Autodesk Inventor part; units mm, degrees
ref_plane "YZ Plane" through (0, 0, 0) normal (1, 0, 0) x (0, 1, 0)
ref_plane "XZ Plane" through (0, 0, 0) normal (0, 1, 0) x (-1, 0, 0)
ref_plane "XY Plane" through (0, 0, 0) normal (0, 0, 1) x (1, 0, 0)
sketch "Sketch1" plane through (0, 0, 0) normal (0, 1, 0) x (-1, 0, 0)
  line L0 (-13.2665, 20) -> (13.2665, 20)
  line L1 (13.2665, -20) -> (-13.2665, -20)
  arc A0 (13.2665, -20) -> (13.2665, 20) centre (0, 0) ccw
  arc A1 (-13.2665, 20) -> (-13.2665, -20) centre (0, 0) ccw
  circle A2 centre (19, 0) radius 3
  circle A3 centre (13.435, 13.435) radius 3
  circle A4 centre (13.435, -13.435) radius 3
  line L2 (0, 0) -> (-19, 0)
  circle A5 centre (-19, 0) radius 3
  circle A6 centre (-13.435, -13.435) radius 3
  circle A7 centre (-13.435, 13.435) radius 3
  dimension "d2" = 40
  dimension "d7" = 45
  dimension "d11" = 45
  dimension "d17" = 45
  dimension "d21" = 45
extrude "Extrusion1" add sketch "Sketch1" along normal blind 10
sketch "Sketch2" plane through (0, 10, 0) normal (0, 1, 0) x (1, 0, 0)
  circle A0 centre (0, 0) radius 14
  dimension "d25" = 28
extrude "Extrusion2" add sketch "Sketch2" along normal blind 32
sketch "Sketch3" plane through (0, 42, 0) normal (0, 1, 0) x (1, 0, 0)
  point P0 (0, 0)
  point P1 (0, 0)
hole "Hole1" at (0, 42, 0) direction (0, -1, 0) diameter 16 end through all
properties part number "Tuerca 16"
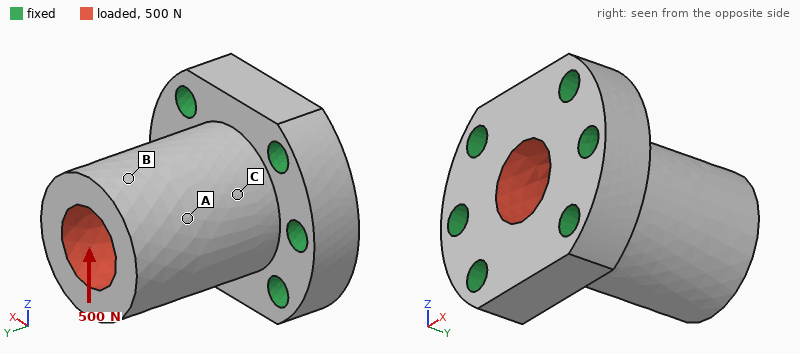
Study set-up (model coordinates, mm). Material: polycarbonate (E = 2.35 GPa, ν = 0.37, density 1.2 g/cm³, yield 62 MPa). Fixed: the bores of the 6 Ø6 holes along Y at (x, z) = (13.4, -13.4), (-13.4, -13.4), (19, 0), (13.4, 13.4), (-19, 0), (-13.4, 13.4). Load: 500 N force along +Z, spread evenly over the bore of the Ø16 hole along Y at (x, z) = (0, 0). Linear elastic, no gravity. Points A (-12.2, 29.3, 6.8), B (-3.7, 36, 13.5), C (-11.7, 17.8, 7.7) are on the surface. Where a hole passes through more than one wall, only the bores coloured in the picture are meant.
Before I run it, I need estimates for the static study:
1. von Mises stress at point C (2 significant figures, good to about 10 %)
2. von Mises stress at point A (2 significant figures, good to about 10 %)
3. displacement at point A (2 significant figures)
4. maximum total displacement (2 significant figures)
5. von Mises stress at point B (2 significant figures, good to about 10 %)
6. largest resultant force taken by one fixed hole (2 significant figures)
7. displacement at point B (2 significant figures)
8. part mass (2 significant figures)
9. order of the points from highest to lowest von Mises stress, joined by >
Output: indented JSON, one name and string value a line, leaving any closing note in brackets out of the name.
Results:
{
  "von Mises stress at point C": "1.6 MPa",
  "von Mises stress at point A": "0.92 MPa",
  "displacement at point A": "56 µm",
  "maximum total displacement": "90 µm",
  "von Mises stress at point B": "0.43 MPa",
  "largest resultant force taken by one fixed hole": "190 N",
  "displacement at point B": "77 µm",
  "part mass": "31 g",
  "order of the points from highest to lowest von Mises stress, joined by >": "C > A > B"
}
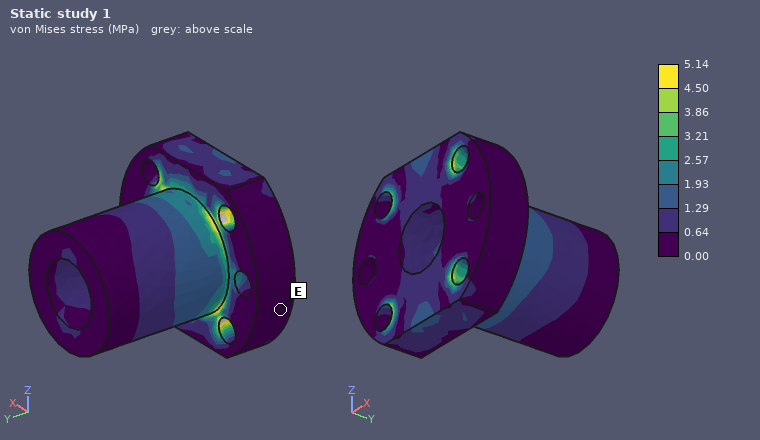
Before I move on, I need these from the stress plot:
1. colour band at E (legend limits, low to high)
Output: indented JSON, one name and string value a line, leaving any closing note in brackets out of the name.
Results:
{
  "colour band at E": "0.00 to 0.64 MPa"
}
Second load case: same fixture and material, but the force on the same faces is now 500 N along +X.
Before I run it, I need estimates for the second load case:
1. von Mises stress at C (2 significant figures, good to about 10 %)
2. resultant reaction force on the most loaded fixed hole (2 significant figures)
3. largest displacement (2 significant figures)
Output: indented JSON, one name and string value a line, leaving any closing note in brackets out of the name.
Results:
{
  "von Mises stress at C": "1.6 MPa",
  "resultant reaction force on the most loaded fixed hole": "160 N",
  "largest displacement": "76 µm"
}
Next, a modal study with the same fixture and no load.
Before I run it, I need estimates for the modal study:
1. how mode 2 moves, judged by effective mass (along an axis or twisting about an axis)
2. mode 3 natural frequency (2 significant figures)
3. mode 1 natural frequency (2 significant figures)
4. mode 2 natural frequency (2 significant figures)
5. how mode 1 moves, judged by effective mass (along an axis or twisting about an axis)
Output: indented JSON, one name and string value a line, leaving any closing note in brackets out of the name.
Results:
{
  "how mode 2 moves, judged by effective mass": "along X",
  "mode 3 natural frequency": "6000 Hz",
  "mode 1 natural frequency": "3100 Hz",
  "mode 2 natural frequency": "3300 Hz",
  "how mode 1 moves, judged by effective mass": "along Z"
}
